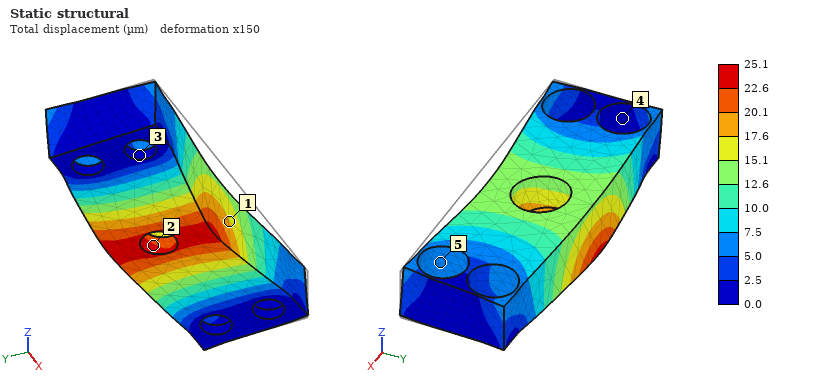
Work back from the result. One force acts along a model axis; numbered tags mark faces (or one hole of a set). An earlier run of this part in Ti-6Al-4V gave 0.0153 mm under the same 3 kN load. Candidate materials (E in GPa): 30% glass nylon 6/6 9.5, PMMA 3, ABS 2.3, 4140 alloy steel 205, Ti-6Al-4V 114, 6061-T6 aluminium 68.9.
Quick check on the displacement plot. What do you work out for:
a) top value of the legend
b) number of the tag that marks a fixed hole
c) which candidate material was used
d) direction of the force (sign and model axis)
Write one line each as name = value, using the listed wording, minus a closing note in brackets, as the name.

top value of the legend = 25.1 µm
number of the tag that marks a fixed hole = 3
which candidate material was used = 6061-T6 aluminium
direction of the force = +Y
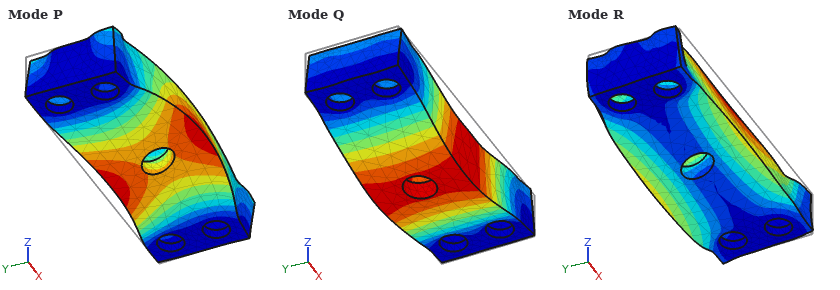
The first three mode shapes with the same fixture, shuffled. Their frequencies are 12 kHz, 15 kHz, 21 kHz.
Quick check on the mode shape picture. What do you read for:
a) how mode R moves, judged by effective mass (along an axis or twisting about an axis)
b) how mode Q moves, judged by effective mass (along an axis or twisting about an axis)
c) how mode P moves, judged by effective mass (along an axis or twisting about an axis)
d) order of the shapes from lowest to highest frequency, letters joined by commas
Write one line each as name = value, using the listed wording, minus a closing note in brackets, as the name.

how mode R moves, judged by effective mass = along Y
how mode Q moves, judged by effective mass = along Z
how mode P moves, judged by effective mass = along Y
order of the shapes from lowest to highest frequency, letters joined by commas = Q, R, P
